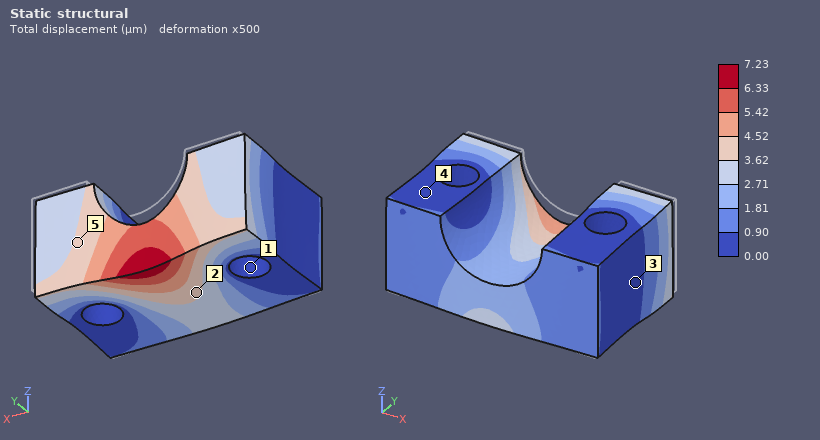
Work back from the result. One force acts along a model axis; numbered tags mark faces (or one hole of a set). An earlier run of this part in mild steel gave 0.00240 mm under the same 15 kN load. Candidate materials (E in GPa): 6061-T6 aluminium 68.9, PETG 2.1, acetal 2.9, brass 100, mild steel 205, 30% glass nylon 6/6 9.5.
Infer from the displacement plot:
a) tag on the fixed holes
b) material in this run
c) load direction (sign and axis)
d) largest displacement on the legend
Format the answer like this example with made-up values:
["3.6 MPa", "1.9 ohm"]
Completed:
["1", "6061-T6 aluminium", "-Y", "7.23 µm"]
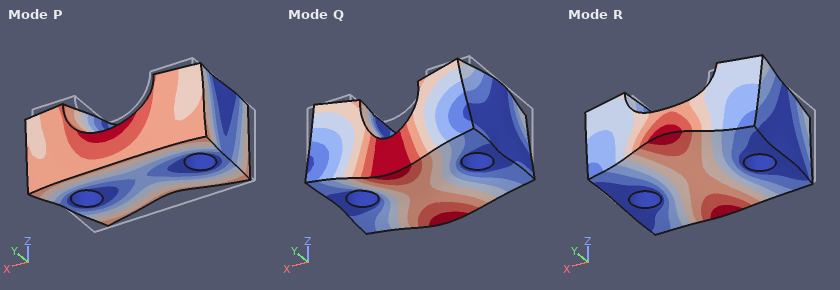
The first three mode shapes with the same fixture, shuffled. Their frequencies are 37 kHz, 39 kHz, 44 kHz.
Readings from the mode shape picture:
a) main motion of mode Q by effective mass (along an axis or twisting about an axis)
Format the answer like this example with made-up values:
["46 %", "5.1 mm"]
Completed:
["along Z"]
